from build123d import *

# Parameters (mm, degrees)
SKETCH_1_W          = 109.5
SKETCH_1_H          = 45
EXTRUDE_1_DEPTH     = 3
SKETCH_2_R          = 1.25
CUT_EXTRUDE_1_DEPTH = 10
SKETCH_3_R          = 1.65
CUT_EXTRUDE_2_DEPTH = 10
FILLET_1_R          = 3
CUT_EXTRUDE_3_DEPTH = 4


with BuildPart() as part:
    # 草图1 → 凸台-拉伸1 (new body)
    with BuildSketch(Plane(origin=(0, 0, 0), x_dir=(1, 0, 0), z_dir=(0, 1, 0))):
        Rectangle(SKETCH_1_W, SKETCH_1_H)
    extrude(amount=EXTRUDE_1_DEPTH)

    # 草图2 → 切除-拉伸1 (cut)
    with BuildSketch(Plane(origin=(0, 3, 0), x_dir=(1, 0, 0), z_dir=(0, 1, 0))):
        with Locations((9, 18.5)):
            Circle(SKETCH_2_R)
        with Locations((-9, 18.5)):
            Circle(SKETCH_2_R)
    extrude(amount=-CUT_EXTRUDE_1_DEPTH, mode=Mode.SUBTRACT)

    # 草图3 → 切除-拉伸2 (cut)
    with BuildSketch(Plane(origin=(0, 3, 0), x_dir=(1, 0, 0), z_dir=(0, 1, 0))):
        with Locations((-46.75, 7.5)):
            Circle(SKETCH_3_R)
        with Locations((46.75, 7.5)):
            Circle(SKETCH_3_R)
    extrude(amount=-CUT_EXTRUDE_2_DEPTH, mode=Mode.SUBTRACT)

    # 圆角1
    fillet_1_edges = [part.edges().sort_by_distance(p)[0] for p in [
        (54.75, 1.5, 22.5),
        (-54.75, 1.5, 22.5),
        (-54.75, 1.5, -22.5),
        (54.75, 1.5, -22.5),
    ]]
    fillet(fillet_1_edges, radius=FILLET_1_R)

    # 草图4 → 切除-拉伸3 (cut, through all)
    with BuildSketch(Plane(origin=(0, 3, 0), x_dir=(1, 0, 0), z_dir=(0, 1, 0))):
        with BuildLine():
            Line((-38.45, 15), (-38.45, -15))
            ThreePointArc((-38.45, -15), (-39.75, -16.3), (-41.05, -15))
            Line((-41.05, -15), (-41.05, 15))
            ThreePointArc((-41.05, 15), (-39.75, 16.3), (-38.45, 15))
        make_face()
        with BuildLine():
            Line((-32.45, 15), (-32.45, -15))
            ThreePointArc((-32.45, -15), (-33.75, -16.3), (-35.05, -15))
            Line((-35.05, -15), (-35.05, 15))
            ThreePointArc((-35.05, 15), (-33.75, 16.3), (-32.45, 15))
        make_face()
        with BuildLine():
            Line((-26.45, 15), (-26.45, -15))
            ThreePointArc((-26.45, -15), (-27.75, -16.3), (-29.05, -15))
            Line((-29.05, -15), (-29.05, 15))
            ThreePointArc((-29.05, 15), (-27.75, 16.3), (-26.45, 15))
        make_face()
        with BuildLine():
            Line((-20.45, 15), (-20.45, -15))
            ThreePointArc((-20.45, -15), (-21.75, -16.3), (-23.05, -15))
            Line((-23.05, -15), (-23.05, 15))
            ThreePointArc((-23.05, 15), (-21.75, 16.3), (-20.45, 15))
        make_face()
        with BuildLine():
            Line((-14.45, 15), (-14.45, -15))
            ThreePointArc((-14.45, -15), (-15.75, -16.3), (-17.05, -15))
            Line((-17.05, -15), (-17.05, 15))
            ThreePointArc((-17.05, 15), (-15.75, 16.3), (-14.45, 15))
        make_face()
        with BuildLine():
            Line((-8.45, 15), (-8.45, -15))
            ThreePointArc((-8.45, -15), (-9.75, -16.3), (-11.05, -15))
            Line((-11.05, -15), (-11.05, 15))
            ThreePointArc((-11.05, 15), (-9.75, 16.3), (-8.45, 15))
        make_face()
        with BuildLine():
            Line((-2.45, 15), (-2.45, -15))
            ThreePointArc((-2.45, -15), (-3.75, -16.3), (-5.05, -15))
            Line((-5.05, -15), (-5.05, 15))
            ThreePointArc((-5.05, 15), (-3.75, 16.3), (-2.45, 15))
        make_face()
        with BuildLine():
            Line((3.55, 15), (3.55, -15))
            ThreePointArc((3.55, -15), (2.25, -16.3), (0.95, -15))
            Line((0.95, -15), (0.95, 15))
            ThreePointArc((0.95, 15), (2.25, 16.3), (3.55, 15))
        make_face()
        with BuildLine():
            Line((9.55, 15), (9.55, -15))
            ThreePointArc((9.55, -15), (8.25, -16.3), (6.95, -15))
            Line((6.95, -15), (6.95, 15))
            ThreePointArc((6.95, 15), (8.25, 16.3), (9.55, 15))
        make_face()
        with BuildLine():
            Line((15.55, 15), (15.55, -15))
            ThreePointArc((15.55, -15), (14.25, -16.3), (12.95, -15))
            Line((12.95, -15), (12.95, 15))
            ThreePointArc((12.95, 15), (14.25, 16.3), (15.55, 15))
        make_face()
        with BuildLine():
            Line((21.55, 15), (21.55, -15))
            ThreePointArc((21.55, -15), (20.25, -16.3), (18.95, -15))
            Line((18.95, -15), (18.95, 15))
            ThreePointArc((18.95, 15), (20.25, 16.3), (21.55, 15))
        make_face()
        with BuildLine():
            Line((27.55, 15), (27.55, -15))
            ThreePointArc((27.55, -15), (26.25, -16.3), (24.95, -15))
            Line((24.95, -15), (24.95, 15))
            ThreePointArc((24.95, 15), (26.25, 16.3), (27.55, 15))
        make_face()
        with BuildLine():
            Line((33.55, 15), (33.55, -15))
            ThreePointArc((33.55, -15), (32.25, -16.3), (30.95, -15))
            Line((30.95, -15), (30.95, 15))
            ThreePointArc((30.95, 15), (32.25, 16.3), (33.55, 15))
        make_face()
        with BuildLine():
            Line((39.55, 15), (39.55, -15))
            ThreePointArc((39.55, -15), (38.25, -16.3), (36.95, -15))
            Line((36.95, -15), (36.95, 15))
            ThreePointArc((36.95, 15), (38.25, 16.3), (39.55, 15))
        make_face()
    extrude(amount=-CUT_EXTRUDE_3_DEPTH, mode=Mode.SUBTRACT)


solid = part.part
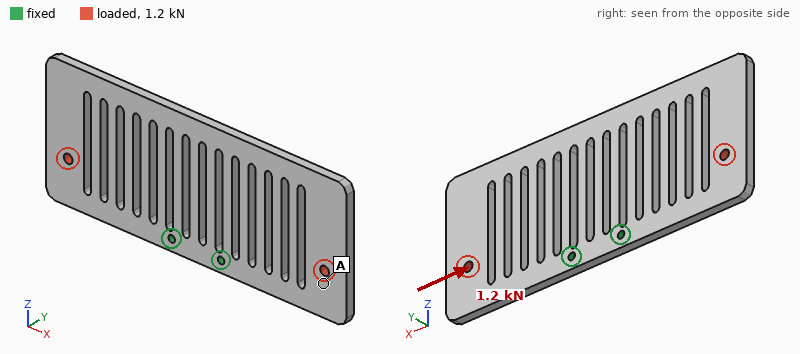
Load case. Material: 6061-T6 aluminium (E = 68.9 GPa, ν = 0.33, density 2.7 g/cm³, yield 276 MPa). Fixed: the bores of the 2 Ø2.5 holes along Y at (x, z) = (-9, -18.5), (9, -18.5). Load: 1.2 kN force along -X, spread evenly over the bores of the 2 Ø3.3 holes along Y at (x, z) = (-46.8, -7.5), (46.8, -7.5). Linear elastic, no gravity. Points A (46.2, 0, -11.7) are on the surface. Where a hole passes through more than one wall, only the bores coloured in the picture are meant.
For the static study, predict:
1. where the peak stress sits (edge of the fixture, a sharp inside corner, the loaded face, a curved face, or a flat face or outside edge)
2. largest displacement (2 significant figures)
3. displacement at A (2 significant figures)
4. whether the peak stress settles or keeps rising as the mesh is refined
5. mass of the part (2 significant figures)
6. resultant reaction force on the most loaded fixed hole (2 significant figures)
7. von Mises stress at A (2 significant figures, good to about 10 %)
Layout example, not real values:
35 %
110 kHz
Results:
edge of the fixture
0.37 mm
0.20 mm
keeps rising
30 g
810 N
25 MPa
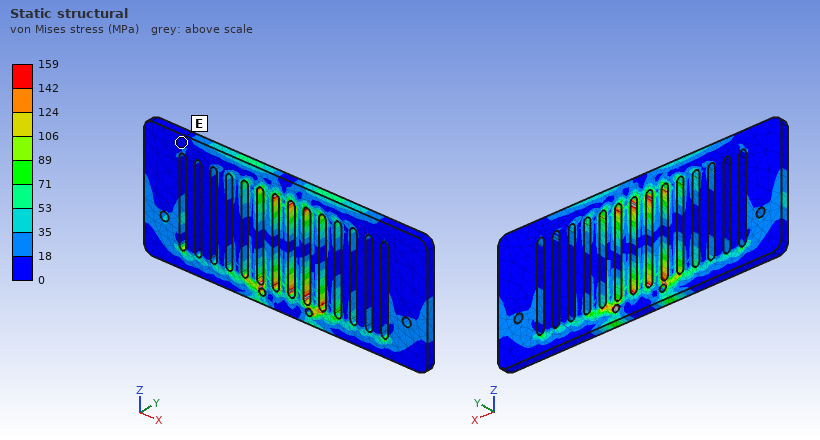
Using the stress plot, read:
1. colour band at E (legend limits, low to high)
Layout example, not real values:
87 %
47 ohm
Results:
0 to 18 MPa
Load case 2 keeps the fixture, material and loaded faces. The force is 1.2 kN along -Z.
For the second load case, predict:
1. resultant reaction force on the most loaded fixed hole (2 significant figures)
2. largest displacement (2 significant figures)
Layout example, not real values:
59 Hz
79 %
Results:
640 N
0.20 mm
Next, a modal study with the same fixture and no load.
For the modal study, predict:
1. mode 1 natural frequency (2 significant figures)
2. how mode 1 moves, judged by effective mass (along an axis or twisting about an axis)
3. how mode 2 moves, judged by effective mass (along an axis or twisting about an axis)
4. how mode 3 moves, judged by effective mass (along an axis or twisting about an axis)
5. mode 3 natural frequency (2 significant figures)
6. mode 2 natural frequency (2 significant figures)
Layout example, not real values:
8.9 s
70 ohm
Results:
490 Hz
twisting about Z
along Y
twisting about X
1100 Hz
530 Hz
